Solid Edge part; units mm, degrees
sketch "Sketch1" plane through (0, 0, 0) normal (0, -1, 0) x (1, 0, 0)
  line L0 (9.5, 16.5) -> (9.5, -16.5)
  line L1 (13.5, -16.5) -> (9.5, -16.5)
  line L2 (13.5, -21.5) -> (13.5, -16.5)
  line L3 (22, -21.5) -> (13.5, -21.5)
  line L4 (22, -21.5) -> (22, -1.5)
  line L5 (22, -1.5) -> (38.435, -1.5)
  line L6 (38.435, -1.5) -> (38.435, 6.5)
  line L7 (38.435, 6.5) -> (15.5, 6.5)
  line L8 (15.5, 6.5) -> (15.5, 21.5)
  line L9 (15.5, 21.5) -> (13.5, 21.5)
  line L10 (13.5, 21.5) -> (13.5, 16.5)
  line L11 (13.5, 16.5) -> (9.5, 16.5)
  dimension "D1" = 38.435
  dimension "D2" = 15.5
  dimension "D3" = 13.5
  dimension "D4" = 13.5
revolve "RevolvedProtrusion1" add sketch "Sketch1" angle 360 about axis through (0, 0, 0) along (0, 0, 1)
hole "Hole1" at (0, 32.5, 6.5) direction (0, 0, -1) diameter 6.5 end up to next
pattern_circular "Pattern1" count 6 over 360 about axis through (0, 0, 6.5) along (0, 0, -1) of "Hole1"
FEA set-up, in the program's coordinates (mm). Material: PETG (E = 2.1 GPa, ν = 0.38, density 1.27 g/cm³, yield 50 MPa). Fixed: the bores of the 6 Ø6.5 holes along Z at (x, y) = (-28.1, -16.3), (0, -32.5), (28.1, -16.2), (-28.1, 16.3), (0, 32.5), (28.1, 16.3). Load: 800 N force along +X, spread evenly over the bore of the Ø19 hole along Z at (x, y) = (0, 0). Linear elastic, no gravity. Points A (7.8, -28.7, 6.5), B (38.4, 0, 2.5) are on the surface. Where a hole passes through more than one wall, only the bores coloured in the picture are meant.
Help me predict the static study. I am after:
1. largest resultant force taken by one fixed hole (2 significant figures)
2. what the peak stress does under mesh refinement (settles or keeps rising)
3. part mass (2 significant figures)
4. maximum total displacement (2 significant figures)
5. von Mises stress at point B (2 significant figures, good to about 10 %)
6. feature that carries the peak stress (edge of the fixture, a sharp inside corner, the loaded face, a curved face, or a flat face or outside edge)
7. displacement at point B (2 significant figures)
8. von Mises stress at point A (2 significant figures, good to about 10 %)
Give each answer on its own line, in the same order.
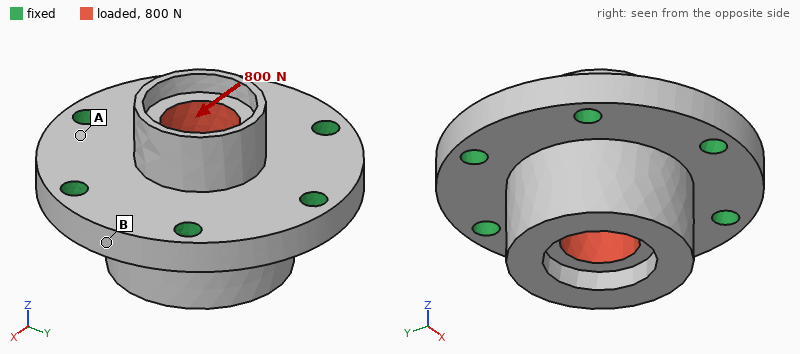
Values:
180 N
keeps rising
79 g
21 µm
0.70 MPa
edge of the fixture
6.9 µm
0.32 MPa
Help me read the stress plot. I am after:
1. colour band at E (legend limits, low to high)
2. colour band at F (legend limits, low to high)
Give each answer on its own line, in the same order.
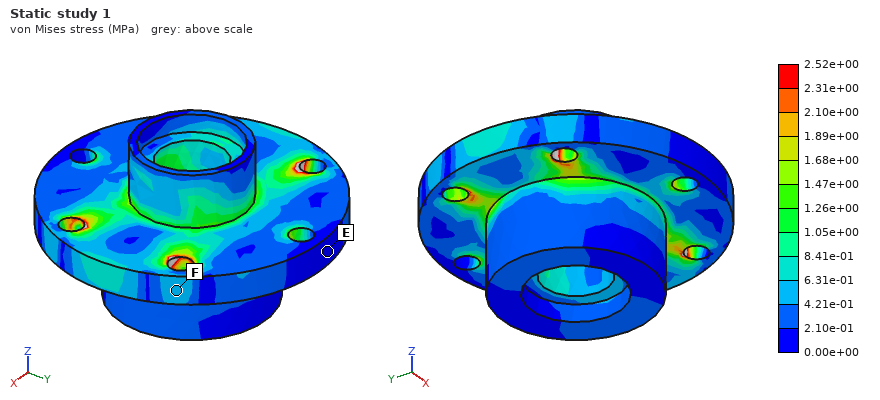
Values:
0.00e+00 to 2.10e-01 MPa
4.21e-01 to 6.31e-01 MPa
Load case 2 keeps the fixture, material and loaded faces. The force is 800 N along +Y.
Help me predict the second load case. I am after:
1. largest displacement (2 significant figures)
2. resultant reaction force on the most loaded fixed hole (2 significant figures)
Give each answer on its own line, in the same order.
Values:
21 µm
200 N
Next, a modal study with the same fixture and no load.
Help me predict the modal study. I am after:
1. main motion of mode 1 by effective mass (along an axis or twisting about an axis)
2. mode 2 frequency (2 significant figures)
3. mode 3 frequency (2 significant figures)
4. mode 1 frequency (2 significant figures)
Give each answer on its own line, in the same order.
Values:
along Z
4000 Hz
4000 Hz
3600 Hz
